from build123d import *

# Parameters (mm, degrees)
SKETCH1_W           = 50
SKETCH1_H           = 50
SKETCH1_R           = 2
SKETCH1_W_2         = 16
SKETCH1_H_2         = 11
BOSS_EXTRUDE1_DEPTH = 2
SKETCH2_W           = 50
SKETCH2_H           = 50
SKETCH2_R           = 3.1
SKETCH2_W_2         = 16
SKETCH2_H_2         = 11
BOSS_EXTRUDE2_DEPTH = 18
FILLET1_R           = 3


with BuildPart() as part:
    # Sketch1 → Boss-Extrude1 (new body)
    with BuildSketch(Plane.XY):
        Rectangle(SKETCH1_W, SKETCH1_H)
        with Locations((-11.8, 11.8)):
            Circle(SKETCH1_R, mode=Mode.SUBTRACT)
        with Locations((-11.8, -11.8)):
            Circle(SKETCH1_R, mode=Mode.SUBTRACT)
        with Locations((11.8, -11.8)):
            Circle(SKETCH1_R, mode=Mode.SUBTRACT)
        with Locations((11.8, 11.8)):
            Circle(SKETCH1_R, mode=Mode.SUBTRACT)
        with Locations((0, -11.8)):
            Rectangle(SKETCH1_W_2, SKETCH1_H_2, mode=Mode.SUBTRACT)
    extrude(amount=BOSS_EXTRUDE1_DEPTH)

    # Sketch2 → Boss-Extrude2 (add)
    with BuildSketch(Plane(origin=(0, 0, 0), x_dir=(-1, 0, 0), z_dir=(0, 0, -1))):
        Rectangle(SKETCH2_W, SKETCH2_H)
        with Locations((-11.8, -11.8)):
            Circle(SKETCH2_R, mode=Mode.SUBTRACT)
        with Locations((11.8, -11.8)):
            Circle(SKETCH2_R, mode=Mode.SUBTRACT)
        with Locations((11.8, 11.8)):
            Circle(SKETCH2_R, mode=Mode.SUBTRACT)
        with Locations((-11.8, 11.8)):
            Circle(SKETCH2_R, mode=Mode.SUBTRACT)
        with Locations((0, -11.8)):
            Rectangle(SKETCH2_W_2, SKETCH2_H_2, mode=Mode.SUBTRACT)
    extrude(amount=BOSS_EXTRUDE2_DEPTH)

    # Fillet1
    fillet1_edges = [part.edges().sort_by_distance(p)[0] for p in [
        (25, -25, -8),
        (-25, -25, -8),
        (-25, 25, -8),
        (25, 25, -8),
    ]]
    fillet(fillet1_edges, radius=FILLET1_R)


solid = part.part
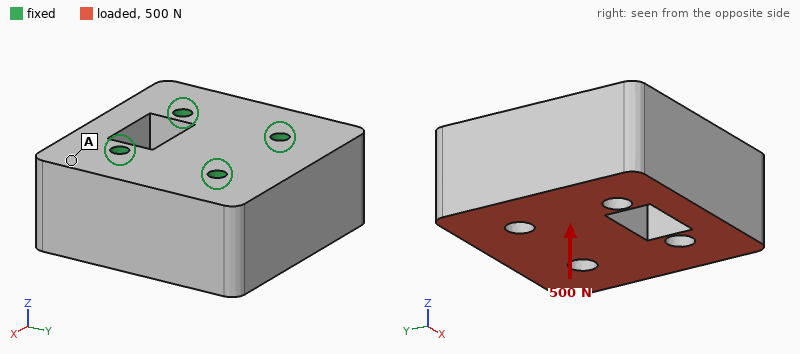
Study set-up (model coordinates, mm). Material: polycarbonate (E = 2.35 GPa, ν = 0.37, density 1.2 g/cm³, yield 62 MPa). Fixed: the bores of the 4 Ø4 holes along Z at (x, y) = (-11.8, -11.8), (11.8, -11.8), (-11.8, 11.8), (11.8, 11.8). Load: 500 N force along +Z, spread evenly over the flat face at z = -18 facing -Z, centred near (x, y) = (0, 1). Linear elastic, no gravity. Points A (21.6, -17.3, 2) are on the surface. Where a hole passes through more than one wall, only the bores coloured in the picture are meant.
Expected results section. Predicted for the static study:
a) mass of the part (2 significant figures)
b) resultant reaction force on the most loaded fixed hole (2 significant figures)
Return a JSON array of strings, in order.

["53 g", "140 N"]
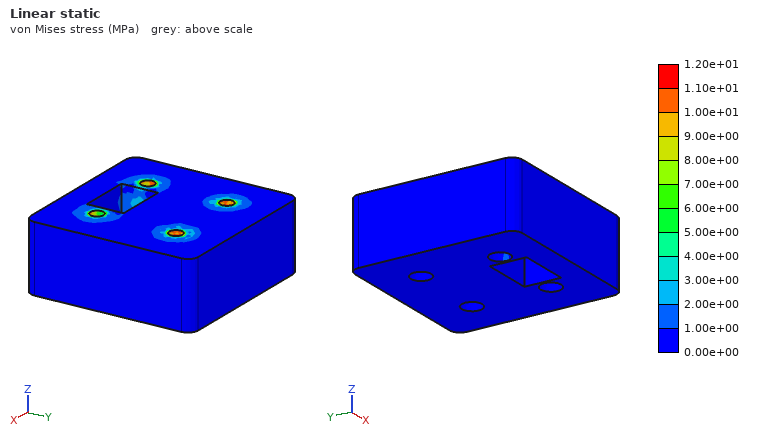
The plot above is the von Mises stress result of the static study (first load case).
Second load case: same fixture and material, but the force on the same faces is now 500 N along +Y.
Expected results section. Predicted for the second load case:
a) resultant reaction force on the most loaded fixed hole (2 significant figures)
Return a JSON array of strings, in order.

["230 N"]
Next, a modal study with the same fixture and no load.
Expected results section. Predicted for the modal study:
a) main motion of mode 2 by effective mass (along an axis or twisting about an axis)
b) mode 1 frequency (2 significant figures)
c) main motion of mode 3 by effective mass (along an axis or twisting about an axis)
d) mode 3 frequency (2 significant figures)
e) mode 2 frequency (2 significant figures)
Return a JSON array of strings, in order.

["along Y", "2400 Hz", "twisting about Z", "3800 Hz", "2500 Hz"]
